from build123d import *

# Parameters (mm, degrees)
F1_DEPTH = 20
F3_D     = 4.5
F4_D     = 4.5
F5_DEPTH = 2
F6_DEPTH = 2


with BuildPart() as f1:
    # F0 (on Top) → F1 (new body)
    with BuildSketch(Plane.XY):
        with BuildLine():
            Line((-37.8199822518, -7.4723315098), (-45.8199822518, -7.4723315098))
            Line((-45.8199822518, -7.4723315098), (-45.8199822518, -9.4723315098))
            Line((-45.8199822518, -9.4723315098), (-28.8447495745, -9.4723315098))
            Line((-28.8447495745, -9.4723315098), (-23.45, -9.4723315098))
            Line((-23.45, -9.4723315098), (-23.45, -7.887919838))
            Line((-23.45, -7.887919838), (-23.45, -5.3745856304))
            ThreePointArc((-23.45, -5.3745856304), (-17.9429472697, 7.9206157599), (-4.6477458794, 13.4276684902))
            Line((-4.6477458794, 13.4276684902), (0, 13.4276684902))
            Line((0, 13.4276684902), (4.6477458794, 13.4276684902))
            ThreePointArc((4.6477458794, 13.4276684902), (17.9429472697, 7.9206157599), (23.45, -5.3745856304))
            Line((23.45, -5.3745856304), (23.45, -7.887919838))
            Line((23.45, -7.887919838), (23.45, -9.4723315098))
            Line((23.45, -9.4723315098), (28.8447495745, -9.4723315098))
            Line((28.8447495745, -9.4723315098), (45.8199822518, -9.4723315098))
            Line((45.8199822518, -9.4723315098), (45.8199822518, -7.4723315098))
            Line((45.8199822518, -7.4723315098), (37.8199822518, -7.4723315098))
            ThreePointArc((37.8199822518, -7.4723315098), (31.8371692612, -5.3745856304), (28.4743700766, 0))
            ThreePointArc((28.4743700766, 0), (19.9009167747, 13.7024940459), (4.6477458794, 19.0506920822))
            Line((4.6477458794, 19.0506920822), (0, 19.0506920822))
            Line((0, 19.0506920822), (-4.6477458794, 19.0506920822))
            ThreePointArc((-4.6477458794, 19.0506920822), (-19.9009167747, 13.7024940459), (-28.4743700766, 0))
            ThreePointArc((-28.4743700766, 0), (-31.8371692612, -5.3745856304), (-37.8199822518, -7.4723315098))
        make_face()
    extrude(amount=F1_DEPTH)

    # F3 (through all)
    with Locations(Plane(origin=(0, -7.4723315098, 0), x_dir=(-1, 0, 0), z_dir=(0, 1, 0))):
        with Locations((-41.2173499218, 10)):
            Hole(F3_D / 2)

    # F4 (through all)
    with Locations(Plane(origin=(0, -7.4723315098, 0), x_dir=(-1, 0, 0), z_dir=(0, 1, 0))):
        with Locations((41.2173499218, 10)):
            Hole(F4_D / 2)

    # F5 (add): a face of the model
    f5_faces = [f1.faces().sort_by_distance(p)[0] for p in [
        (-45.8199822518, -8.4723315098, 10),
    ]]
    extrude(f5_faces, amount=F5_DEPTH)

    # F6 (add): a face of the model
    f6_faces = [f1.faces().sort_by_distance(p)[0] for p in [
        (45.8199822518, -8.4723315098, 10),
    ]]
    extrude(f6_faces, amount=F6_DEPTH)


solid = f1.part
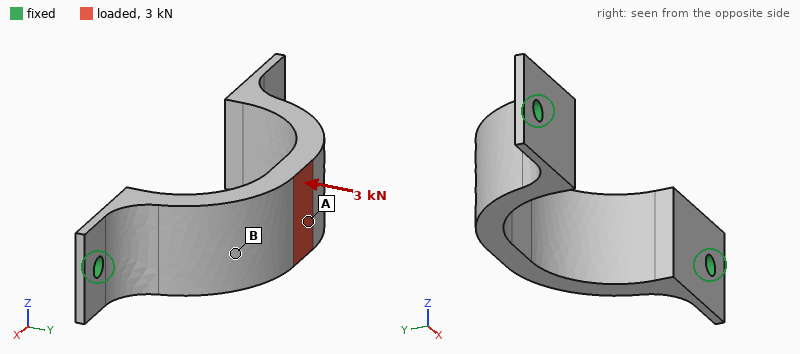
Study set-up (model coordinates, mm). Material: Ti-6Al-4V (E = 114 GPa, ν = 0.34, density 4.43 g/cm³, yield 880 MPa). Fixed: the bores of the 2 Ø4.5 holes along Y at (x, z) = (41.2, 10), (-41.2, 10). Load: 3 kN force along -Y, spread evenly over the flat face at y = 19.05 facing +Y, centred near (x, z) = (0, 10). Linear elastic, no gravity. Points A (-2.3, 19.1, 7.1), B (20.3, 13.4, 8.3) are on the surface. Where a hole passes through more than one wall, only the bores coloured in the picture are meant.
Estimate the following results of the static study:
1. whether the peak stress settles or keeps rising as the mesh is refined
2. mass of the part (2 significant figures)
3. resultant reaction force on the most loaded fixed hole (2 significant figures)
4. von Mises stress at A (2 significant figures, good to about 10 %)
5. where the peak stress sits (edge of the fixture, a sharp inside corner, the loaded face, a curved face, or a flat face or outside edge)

keeps rising
51 g
2.3 kN
86 MPa
edge of the fixture
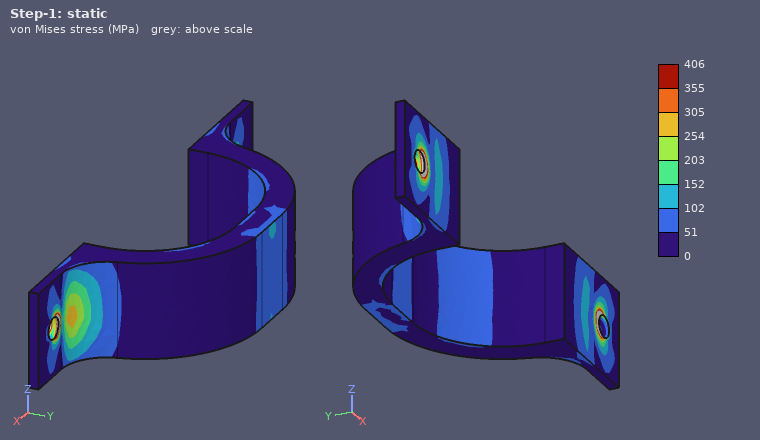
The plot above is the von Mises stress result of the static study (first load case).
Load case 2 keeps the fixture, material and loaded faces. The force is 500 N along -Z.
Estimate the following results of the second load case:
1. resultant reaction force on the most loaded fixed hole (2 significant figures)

250 N
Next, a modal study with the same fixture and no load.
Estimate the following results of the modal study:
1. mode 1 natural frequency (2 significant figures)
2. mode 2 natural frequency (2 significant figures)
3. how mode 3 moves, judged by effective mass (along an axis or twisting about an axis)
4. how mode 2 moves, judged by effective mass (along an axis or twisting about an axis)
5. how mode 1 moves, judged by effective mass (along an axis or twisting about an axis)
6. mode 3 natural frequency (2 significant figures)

1300 Hz
4800 Hz
along Y
along X
along Z
5100 Hz
